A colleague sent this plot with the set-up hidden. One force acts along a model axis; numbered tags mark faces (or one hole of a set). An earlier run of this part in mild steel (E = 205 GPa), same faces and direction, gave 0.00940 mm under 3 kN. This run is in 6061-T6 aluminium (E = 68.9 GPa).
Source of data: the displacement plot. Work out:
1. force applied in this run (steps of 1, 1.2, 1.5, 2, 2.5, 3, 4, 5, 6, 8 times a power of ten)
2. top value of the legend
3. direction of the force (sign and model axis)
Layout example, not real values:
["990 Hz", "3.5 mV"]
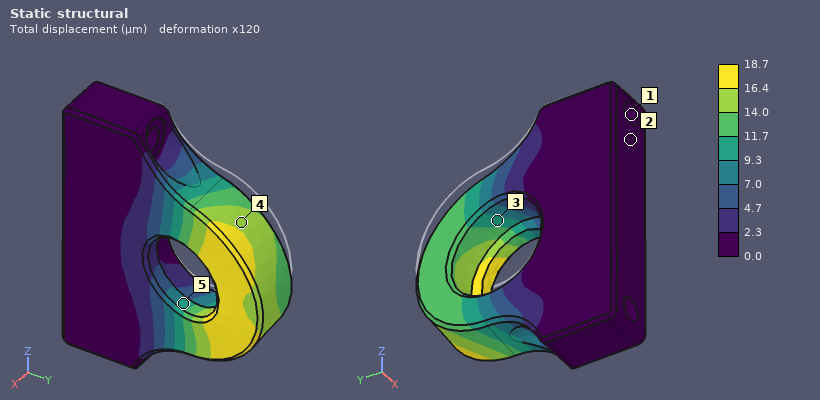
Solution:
["2 kN", "18.7 µm", "-Z"]
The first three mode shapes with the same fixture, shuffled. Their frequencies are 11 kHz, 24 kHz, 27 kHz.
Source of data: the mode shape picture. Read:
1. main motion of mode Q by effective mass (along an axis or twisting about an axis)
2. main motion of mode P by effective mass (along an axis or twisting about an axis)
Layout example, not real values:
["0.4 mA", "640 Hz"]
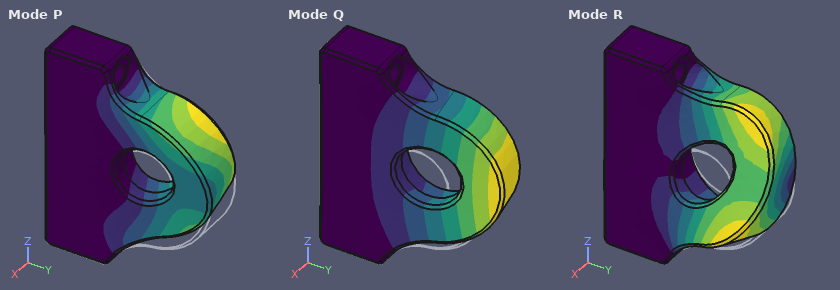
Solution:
["along X", "along Z"]
